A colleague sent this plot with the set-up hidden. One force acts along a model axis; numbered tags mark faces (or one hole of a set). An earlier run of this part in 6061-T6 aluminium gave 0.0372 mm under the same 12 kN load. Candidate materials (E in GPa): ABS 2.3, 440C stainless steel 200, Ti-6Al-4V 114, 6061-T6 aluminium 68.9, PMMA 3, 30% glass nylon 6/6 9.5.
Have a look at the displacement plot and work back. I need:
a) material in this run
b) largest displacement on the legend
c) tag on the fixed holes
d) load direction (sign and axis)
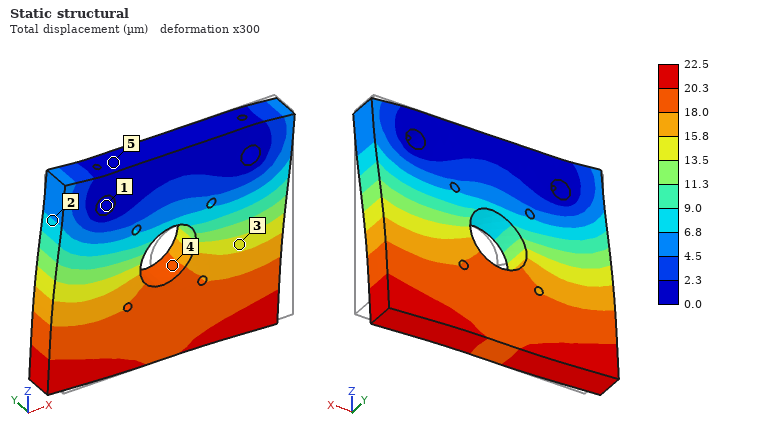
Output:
Ti-6Al-4V
22.5 µm
1
-X
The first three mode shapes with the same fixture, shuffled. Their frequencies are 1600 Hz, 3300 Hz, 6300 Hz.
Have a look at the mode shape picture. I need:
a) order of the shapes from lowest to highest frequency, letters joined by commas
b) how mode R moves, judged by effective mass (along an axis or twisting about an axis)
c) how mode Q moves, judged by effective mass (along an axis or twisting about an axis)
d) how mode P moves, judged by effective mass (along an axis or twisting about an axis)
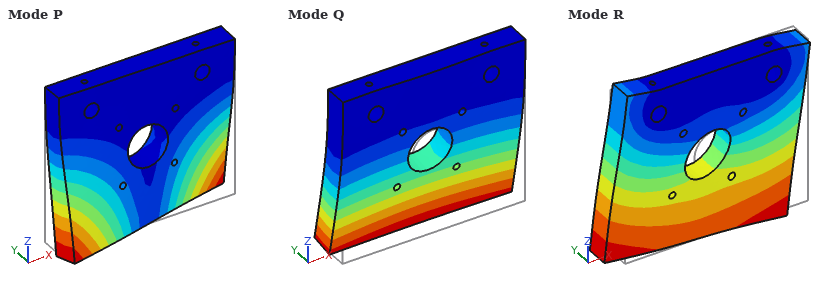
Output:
Q, P, R
along X
along Y
twisting about Z
